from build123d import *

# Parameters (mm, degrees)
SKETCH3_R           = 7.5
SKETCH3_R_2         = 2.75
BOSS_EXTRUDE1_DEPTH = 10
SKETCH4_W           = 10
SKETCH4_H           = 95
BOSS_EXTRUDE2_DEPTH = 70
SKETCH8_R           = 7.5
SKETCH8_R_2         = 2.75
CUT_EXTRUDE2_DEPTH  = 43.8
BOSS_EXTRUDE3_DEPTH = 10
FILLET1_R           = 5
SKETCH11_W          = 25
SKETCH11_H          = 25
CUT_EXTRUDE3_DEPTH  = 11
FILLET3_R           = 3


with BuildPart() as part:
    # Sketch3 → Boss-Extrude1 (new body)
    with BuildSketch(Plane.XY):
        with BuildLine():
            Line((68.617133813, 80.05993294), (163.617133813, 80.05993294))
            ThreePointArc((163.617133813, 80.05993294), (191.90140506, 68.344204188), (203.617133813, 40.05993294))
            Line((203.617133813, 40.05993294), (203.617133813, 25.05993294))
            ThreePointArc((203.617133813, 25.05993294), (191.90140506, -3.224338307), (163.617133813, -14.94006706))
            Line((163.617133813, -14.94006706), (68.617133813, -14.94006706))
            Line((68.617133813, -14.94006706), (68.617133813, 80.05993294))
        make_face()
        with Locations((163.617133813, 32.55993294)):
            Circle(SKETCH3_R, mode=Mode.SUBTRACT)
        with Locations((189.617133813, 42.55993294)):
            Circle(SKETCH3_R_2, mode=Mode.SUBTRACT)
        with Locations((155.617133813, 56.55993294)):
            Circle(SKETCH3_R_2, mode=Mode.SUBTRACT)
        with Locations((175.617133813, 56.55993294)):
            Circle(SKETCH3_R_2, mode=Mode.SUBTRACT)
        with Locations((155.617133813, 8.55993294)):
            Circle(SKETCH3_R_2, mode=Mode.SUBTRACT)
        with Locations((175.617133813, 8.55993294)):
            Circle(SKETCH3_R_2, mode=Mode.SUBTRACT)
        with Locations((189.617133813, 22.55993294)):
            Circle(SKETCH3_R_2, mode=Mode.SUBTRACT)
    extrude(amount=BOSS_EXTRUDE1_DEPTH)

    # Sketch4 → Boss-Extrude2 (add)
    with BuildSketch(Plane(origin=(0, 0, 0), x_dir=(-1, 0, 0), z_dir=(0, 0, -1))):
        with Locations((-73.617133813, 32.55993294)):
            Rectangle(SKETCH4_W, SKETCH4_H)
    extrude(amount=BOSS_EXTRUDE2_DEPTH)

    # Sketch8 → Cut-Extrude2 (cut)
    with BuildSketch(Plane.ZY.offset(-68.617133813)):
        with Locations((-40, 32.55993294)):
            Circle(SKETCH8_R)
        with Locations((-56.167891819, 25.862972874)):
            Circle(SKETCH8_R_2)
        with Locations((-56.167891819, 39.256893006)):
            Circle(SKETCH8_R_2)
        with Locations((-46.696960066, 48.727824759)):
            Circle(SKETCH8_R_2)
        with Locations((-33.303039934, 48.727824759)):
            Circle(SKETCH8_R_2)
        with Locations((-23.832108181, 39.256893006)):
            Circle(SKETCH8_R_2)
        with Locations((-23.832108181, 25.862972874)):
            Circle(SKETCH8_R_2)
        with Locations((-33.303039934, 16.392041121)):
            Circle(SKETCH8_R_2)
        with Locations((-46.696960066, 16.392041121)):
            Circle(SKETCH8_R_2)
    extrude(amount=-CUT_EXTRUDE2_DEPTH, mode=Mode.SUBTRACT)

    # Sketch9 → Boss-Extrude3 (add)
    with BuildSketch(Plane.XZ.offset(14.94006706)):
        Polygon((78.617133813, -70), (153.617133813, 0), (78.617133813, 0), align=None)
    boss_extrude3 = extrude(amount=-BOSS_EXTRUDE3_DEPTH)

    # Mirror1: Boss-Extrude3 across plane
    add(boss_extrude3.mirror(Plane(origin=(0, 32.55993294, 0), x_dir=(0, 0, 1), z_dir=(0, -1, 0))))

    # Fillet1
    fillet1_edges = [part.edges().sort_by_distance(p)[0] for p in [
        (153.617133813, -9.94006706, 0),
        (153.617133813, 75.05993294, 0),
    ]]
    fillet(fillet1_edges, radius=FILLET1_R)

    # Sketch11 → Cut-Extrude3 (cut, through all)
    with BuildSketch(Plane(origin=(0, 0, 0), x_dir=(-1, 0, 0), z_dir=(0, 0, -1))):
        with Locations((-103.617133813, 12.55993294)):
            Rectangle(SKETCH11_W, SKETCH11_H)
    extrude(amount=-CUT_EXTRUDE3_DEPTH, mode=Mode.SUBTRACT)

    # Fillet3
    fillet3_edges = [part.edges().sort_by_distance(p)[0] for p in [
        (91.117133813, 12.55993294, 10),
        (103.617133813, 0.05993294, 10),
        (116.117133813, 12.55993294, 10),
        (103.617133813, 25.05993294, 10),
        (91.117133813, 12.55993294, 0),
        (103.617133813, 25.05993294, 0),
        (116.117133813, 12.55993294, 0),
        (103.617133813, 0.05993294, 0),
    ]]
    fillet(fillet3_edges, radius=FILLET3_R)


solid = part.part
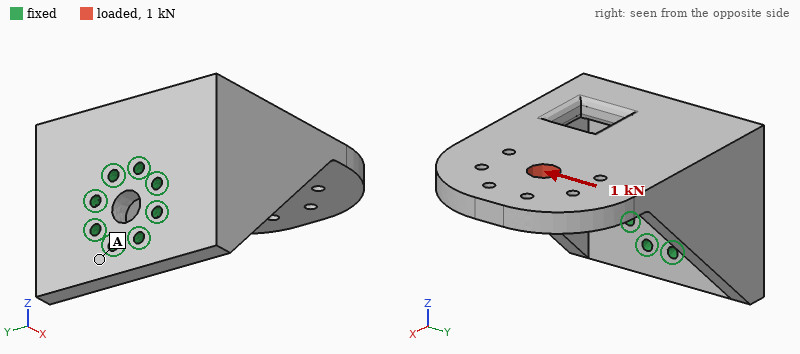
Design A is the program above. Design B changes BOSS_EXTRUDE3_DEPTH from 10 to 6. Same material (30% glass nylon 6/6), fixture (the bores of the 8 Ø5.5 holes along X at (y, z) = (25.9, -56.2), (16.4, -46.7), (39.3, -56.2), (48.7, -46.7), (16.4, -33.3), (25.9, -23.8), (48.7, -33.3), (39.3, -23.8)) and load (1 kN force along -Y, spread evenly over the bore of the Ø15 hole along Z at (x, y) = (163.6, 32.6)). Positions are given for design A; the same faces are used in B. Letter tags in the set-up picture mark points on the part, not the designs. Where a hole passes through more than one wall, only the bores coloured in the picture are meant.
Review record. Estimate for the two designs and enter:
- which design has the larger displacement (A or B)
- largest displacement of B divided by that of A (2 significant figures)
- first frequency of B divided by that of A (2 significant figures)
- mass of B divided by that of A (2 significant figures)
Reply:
B
1.2
0.94
0.91
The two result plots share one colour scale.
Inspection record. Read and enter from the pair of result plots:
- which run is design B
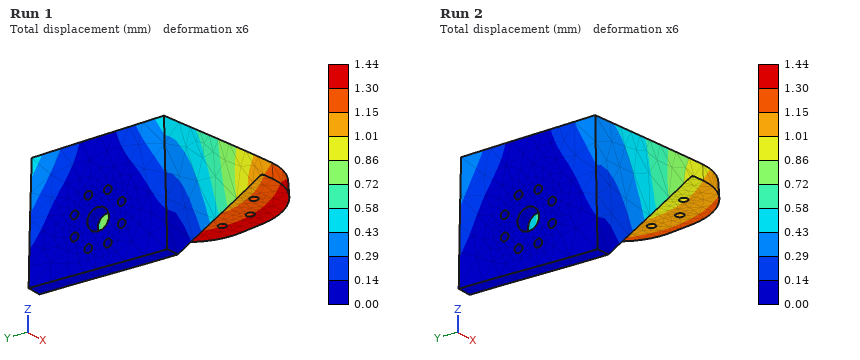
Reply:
Run 1
